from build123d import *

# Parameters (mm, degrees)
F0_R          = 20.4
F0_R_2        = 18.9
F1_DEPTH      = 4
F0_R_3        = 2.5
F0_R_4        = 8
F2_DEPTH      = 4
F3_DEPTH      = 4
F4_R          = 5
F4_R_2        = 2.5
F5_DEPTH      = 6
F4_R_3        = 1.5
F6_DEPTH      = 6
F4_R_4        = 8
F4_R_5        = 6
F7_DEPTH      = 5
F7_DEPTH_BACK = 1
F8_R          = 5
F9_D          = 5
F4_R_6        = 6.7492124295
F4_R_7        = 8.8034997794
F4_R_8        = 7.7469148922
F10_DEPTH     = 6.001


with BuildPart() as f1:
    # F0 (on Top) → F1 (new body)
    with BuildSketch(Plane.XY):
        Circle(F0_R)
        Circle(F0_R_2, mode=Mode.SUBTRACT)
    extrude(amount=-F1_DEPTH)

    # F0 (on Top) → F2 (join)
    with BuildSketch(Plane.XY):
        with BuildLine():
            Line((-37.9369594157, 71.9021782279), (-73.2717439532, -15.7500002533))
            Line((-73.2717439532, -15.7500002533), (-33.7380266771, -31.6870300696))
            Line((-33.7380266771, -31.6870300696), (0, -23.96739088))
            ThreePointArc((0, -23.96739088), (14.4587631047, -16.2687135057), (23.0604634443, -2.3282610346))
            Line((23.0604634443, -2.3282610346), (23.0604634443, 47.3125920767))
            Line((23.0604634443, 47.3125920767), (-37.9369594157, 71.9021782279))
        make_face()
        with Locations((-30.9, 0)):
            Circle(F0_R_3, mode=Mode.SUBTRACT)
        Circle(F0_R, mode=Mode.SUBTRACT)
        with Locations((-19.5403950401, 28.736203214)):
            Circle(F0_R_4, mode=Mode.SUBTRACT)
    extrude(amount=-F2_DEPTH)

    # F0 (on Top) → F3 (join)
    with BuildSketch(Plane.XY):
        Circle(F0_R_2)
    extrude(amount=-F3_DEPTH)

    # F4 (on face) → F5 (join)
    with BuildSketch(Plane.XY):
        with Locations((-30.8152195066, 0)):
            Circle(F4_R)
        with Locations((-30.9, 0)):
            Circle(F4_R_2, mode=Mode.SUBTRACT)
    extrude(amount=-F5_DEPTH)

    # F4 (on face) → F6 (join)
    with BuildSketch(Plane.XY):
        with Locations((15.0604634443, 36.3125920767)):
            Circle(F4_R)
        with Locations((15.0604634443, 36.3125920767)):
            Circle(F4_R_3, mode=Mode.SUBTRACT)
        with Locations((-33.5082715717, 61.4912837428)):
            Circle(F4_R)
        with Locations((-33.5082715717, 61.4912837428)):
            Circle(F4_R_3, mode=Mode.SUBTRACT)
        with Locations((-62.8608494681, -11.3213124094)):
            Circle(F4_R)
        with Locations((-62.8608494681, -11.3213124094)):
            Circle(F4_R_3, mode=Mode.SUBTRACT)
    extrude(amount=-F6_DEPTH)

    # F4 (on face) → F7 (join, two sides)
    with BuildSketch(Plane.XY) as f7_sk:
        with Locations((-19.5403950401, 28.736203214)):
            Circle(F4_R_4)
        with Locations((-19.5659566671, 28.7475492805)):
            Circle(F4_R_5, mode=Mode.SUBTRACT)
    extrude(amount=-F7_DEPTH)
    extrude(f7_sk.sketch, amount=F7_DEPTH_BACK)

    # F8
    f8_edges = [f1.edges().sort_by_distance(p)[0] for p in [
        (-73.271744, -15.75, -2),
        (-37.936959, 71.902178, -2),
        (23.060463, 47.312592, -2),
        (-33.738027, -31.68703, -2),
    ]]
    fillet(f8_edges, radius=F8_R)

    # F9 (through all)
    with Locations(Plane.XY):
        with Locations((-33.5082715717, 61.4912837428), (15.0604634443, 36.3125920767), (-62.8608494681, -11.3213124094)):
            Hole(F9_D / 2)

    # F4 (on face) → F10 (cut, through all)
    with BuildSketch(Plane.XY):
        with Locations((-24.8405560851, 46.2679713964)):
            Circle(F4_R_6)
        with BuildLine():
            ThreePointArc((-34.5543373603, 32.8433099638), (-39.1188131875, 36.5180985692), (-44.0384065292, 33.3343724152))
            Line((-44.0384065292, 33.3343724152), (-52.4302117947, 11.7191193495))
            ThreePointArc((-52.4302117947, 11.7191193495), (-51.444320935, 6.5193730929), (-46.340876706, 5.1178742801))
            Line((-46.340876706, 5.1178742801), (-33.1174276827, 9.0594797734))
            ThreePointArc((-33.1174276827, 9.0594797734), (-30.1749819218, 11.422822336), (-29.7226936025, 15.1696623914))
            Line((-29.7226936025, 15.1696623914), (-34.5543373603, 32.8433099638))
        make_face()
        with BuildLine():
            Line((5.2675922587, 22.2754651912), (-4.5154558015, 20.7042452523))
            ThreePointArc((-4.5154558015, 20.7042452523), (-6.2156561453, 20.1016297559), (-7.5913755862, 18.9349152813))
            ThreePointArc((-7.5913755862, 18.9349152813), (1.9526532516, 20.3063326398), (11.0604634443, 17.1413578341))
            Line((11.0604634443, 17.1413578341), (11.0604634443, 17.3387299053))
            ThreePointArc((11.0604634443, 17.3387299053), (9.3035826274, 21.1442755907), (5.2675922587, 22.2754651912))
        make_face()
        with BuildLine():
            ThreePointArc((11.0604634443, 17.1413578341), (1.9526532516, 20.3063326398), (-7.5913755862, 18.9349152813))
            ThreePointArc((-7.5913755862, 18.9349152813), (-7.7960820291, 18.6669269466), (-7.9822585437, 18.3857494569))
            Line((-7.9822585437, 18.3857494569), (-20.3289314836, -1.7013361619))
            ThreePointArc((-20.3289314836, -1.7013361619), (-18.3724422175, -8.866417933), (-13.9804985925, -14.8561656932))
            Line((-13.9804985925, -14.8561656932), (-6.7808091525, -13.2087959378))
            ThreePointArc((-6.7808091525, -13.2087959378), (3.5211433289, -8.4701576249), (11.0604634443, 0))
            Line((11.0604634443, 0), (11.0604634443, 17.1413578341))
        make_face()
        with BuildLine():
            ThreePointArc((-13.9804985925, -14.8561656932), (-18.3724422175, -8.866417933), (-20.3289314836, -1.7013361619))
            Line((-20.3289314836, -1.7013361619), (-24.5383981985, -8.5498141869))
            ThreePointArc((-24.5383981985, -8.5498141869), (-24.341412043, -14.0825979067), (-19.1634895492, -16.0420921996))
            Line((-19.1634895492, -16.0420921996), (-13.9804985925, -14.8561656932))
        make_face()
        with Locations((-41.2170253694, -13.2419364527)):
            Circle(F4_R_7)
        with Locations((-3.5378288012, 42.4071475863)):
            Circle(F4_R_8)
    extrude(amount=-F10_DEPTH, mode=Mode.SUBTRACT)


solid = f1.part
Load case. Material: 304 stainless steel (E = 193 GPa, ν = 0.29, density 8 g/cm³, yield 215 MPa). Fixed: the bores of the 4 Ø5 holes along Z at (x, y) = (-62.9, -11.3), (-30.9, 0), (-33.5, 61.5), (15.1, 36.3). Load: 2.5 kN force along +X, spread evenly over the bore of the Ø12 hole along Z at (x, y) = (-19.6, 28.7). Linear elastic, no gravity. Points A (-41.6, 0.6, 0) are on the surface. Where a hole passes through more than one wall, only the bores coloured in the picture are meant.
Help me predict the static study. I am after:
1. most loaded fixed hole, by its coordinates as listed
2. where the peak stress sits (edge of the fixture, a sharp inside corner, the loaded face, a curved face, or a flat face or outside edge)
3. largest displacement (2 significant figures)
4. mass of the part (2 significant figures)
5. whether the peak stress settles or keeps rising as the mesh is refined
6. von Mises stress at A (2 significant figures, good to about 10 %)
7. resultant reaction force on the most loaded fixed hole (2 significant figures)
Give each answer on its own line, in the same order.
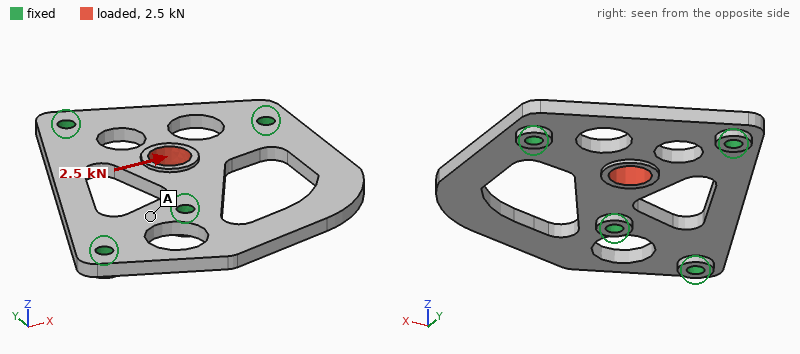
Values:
(15.1, 36.3)
edge of the fixture
6.8 µm
160 g
keeps rising
6.2 MPa
1.3 kN
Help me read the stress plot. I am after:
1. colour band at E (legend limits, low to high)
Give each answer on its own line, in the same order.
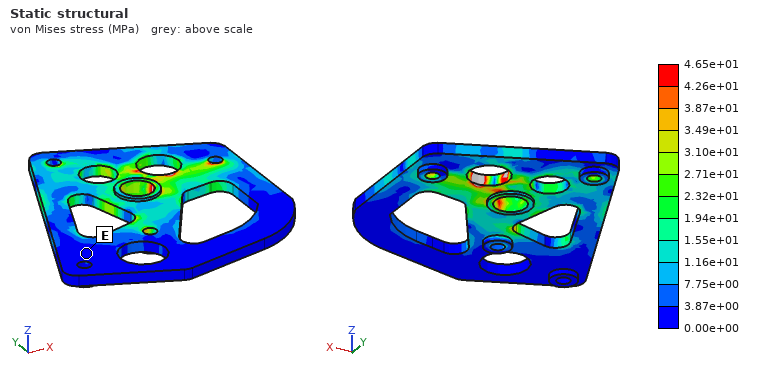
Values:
0.00e+00 to 3.87e+00 MPa
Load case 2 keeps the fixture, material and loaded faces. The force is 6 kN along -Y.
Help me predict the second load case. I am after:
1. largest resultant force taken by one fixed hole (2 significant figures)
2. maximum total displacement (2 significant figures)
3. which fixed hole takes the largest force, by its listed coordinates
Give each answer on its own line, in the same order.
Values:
2.8 kN
12 µm
(-30.9, 0)
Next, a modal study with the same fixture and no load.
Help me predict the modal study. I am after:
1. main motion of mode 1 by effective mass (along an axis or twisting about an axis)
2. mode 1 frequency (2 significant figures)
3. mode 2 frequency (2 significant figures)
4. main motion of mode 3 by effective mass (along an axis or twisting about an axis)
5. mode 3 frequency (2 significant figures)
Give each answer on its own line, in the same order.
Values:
along Z
1600 Hz
3900 Hz
along Z
4700 Hz
